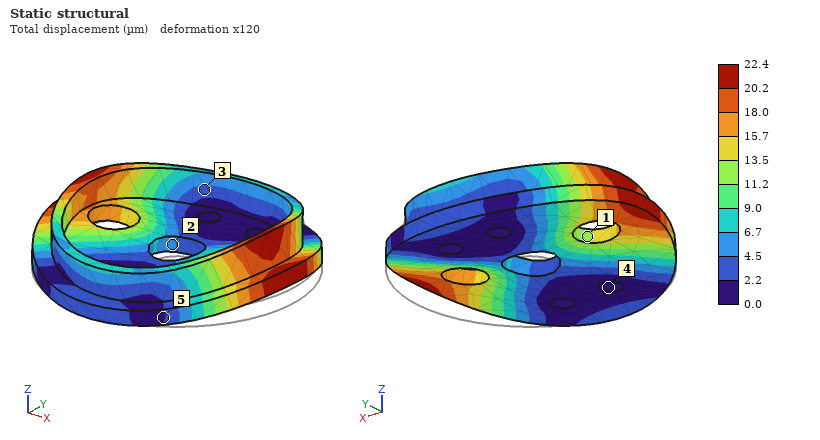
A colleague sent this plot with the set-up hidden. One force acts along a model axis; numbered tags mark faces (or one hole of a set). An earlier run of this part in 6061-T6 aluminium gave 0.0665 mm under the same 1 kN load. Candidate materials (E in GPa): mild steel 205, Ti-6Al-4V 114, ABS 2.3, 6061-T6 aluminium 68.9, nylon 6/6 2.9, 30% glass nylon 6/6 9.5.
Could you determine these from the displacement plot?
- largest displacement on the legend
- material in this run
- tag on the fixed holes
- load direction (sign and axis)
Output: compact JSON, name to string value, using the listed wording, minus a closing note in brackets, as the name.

{"largest displacement on the legend": "22.4 µm", "material in this run": "mild steel", "tag on the fixed holes": "4", "load direction": "+Z"}
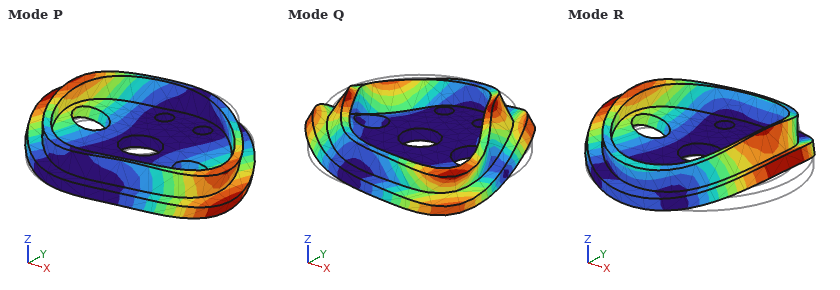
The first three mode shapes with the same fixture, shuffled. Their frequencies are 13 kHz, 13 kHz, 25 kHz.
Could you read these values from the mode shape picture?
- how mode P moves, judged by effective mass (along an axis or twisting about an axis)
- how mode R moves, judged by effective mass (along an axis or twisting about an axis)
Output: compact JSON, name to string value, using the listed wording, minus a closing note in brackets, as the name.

{"how mode P moves, judged by effective mass": "twisting about Y", "how mode R moves, judged by effective mass": "along Z"}
